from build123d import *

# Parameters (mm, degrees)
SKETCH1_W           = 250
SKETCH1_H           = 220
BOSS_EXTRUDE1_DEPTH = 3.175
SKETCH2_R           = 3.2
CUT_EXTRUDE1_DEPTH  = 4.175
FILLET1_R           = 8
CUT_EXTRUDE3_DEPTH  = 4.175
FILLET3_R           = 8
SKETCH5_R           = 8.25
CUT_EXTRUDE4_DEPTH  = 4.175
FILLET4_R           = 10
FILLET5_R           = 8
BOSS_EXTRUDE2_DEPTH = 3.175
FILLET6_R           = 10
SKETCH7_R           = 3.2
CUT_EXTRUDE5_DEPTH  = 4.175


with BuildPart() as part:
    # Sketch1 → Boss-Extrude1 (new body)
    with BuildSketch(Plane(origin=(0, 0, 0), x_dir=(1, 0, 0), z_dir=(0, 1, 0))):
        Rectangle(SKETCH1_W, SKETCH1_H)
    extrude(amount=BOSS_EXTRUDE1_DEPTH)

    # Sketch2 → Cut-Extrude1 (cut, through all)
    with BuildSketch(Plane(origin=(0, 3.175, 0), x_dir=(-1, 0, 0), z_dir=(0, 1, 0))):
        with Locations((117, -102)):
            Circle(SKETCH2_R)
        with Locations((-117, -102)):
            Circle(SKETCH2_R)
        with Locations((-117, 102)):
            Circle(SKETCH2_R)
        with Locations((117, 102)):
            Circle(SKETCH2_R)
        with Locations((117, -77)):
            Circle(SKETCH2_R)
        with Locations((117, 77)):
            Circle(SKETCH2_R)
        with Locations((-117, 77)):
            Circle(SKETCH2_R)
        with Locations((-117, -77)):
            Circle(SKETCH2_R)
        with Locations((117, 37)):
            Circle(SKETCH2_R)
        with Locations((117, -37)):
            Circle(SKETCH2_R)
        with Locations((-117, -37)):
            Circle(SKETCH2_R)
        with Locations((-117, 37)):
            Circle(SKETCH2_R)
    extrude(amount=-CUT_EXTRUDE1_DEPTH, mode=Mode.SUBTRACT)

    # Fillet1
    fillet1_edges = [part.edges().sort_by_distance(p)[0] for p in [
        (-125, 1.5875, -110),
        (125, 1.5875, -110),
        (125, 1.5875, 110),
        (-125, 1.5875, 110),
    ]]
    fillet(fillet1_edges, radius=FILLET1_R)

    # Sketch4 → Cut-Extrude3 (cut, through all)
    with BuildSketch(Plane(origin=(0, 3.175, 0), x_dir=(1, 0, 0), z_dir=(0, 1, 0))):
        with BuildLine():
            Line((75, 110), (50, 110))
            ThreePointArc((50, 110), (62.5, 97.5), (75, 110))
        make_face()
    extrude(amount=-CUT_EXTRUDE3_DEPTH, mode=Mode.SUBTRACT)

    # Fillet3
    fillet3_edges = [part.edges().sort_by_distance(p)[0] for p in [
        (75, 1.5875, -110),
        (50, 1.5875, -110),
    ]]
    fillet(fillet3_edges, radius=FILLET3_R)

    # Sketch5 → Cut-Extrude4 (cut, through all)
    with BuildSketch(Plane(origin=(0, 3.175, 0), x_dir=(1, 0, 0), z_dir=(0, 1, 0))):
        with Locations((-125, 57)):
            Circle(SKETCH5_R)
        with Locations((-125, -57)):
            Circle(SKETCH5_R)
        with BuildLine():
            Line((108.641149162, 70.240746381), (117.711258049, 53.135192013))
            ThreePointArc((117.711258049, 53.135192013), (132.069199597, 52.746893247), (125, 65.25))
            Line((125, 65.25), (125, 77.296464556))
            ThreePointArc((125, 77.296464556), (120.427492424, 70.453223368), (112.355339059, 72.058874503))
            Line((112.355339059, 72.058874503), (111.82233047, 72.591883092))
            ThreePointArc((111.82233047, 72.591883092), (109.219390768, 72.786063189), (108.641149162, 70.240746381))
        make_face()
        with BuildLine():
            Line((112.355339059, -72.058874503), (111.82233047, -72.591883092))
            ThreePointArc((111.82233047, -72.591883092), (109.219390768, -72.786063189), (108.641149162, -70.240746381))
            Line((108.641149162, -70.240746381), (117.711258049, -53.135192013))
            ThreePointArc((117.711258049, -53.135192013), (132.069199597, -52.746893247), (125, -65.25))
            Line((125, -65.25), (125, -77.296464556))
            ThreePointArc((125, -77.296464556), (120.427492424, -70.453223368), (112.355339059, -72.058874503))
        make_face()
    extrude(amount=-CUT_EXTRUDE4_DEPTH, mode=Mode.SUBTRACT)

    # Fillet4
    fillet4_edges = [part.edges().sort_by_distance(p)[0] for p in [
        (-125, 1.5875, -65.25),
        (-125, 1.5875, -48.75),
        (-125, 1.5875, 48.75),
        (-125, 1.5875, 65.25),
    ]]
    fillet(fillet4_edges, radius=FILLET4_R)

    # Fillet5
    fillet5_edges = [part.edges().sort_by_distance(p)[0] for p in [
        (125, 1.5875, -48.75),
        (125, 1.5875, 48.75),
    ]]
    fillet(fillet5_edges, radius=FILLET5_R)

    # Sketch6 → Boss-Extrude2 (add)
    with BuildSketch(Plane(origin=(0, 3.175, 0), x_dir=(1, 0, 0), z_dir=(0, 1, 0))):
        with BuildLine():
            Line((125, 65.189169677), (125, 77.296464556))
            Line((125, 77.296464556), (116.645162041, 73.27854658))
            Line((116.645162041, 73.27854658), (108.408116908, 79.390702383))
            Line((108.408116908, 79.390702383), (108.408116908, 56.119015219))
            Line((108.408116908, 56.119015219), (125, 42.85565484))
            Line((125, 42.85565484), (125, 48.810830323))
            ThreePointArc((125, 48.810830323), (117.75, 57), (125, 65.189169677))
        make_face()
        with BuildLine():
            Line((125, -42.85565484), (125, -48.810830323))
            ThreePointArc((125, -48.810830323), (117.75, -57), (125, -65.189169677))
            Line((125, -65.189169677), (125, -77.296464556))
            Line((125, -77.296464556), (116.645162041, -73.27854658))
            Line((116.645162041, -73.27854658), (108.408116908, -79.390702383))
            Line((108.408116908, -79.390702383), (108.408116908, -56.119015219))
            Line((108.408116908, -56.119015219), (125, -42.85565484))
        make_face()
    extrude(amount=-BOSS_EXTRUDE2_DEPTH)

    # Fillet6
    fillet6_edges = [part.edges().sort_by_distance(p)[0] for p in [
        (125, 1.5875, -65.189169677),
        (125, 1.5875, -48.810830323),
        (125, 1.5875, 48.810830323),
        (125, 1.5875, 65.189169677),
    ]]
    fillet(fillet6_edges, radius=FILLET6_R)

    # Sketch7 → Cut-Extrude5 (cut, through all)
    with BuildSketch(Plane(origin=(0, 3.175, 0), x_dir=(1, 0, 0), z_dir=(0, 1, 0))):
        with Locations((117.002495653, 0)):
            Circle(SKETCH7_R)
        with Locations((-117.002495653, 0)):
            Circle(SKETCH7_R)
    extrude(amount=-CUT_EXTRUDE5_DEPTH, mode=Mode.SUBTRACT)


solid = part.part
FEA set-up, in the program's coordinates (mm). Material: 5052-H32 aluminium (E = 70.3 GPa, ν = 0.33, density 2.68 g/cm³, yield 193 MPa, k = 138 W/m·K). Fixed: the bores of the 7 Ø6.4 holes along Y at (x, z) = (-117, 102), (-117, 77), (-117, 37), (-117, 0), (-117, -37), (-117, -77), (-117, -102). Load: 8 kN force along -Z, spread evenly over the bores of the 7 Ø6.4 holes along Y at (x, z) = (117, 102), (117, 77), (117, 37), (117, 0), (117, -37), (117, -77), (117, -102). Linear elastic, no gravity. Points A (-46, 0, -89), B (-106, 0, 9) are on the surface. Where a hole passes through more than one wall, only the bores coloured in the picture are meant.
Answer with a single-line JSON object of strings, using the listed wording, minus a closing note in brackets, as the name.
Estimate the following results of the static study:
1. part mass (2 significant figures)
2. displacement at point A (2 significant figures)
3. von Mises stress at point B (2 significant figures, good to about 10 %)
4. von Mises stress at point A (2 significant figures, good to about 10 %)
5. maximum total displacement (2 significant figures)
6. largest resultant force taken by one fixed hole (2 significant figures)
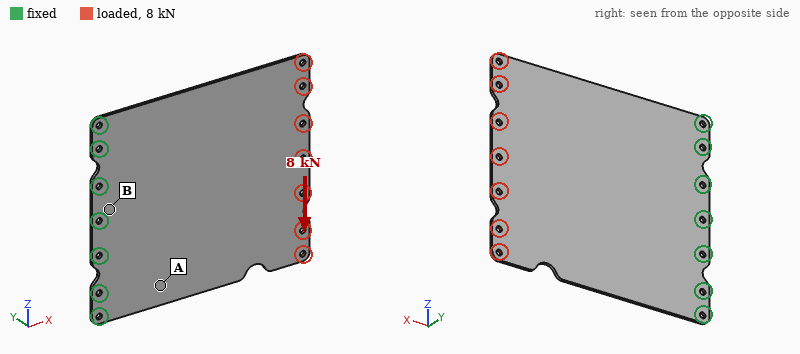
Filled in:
{"part mass": "460 g", "displacement at point A": "0.082 mm", "von Mises stress at point B": "16 MPa", "von Mises stress at point A": "43 MPa", "maximum total displacement": "0.36 mm", "largest resultant force taken by one fixed hole": "5.5 kN"}
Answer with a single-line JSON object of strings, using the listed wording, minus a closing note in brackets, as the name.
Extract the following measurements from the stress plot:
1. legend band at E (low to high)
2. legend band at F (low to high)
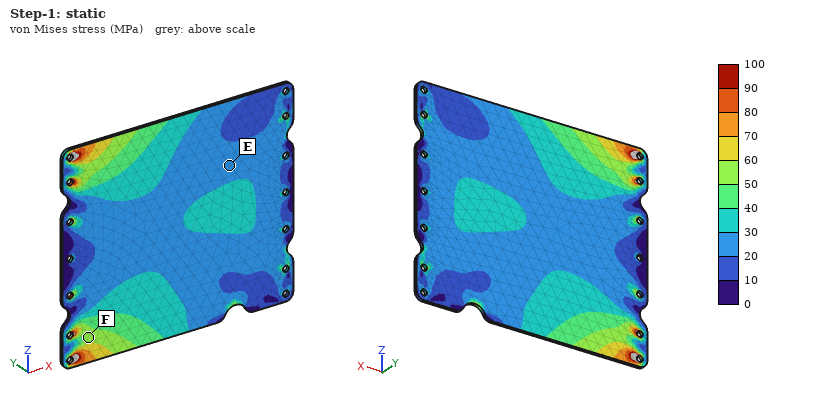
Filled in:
{"legend band at E": "20 to 30 MPa", "legend band at F": "50 to 60 MPa"}
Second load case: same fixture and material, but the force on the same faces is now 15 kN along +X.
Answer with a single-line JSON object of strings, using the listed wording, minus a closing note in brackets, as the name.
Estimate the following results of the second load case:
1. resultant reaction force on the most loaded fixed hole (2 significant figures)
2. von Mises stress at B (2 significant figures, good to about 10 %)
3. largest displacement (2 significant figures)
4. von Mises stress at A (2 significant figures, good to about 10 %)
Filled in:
{"resultant reaction force on the most loaded fixed hole": "2.4 kN", "von Mises stress at B": "19 MPa", "largest displacement": "0.11 mm", "von Mises stress at A": "22 MPa"}
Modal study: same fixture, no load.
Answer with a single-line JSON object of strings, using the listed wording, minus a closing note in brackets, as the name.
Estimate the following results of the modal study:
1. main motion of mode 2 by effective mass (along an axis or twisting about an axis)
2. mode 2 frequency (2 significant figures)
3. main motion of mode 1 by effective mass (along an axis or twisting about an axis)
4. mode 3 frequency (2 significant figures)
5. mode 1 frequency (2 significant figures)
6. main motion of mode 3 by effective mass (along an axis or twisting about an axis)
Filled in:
{"main motion of mode 2 by effective mass": "twisting about X", "mode 2 frequency": "120 Hz", "main motion of mode 1 by effective mass": "along Y", "mode 3 frequency": "290 Hz", "mode 1 frequency": "47 Hz", "main motion of mode 3 by effective mass": "along Y"}
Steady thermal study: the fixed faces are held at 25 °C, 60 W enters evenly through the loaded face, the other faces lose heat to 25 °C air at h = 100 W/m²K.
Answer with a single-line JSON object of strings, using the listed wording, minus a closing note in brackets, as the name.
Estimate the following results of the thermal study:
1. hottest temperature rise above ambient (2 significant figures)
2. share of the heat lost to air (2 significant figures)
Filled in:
{"hottest temperature rise above ambient": "35 K", "share of the heat lost to air": "99 %"}
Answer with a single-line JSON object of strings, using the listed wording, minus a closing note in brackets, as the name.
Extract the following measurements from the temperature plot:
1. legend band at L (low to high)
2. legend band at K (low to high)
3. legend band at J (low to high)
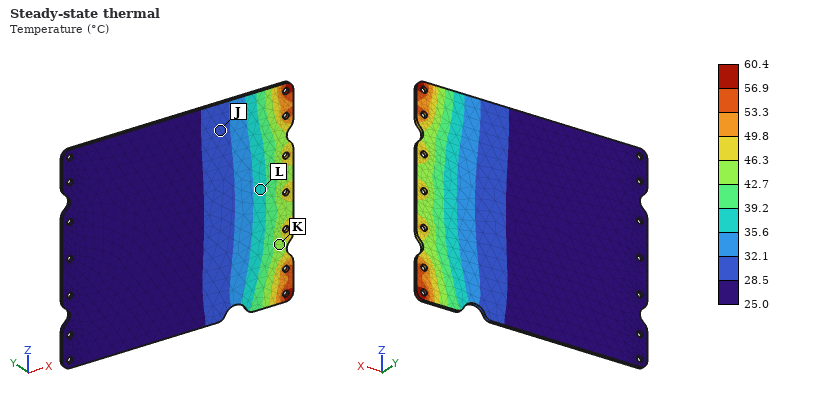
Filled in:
{"legend band at L": "35.6 to 39.2 °C", "legend band at K": "42.7 to 46.3 °C", "legend band at J": "28.5 to 32.1 °C"}
